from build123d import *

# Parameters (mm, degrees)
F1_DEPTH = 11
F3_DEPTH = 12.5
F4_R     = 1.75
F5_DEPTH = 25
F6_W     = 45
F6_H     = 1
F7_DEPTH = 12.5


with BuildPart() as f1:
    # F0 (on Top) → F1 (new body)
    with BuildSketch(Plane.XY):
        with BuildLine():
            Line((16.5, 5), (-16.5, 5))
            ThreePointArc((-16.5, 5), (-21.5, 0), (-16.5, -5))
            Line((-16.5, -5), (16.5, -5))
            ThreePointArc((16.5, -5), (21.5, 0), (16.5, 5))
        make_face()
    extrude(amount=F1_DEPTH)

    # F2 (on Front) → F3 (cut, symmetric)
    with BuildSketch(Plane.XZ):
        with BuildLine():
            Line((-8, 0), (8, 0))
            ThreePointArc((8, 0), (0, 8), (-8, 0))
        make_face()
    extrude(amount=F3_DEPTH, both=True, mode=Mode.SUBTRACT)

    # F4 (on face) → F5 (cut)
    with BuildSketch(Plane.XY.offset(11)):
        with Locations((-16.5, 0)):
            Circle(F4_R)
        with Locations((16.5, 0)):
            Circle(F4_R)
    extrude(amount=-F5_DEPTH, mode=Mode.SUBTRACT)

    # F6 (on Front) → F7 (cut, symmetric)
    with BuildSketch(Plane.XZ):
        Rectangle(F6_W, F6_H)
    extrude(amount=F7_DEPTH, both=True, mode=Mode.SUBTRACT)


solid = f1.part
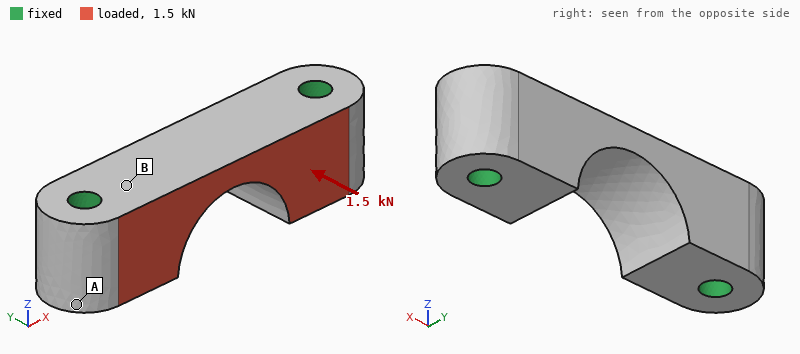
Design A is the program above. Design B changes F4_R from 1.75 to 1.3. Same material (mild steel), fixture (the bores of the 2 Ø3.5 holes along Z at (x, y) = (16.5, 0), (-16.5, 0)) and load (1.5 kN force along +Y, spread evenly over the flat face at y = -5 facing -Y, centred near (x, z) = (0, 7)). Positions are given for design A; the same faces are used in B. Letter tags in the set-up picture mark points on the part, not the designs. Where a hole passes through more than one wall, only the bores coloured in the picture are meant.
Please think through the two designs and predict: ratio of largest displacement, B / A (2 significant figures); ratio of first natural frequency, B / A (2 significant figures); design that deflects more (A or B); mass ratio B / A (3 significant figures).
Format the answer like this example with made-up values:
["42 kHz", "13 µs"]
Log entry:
["1.3", "0.85", "B", "1.03"]
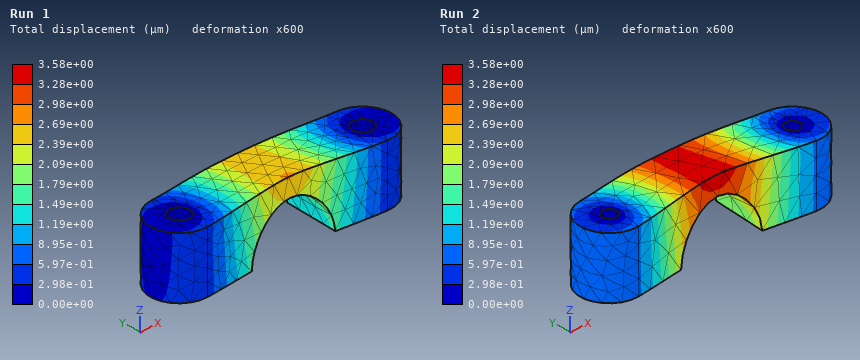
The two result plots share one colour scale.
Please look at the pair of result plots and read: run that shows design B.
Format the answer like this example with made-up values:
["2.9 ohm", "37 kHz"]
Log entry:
["Run 2"]
